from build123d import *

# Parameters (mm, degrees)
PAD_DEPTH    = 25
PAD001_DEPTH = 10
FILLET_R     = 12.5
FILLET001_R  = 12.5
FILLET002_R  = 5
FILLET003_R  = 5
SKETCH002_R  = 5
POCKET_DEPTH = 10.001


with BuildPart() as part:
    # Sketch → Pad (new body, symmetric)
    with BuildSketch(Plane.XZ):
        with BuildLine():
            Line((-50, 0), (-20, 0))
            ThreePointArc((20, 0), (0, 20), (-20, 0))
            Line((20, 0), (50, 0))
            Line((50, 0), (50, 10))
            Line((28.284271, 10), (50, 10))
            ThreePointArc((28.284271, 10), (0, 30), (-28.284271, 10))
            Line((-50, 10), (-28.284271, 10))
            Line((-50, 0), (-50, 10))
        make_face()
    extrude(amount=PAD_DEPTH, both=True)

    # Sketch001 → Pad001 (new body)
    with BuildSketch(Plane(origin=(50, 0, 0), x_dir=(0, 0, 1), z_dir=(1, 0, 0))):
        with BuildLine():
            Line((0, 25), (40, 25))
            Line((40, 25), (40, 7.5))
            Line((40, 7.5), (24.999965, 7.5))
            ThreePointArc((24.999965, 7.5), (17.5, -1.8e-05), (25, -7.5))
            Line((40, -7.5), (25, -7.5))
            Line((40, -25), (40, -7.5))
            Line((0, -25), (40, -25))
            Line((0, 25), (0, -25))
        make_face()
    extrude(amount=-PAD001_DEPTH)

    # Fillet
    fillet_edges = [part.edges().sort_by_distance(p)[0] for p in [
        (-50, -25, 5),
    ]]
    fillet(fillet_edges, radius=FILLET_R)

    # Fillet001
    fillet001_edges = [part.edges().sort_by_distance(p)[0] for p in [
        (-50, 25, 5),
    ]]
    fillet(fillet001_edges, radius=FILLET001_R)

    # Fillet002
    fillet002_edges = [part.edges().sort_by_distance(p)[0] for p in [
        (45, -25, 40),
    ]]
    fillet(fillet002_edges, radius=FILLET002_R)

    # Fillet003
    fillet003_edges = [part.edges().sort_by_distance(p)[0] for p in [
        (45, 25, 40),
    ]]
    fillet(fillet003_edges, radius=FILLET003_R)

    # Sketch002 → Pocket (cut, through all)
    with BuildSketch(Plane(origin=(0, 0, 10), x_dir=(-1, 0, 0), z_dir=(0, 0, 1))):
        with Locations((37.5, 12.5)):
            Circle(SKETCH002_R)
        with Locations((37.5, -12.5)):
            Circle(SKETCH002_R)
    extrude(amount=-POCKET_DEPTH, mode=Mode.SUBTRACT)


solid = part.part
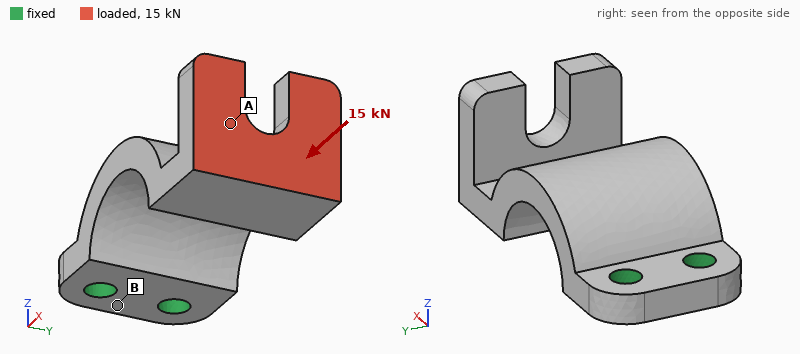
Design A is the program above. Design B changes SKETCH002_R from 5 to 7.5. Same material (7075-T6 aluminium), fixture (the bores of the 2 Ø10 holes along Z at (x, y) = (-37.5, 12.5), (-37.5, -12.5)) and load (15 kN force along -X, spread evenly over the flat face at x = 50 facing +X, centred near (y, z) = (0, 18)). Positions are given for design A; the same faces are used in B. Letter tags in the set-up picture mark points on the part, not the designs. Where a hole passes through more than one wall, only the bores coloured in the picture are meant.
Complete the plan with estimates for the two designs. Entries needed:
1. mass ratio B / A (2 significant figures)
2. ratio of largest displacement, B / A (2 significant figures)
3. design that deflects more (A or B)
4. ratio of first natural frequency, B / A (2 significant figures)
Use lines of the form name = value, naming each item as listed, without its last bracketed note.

mass ratio B / A = 0.97
ratio of largest displacement, B / A = 0.87
design that deflects more = A
ratio of first natural frequency, B / A = 1.1
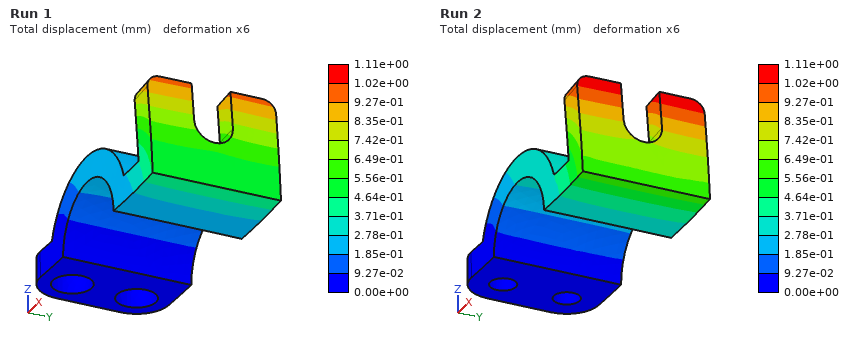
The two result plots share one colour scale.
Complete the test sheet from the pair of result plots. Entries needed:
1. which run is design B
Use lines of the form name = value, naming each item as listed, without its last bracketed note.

which run is design B = Run 1
